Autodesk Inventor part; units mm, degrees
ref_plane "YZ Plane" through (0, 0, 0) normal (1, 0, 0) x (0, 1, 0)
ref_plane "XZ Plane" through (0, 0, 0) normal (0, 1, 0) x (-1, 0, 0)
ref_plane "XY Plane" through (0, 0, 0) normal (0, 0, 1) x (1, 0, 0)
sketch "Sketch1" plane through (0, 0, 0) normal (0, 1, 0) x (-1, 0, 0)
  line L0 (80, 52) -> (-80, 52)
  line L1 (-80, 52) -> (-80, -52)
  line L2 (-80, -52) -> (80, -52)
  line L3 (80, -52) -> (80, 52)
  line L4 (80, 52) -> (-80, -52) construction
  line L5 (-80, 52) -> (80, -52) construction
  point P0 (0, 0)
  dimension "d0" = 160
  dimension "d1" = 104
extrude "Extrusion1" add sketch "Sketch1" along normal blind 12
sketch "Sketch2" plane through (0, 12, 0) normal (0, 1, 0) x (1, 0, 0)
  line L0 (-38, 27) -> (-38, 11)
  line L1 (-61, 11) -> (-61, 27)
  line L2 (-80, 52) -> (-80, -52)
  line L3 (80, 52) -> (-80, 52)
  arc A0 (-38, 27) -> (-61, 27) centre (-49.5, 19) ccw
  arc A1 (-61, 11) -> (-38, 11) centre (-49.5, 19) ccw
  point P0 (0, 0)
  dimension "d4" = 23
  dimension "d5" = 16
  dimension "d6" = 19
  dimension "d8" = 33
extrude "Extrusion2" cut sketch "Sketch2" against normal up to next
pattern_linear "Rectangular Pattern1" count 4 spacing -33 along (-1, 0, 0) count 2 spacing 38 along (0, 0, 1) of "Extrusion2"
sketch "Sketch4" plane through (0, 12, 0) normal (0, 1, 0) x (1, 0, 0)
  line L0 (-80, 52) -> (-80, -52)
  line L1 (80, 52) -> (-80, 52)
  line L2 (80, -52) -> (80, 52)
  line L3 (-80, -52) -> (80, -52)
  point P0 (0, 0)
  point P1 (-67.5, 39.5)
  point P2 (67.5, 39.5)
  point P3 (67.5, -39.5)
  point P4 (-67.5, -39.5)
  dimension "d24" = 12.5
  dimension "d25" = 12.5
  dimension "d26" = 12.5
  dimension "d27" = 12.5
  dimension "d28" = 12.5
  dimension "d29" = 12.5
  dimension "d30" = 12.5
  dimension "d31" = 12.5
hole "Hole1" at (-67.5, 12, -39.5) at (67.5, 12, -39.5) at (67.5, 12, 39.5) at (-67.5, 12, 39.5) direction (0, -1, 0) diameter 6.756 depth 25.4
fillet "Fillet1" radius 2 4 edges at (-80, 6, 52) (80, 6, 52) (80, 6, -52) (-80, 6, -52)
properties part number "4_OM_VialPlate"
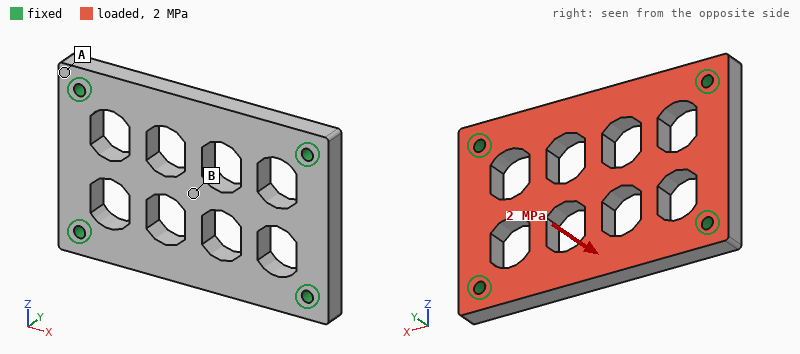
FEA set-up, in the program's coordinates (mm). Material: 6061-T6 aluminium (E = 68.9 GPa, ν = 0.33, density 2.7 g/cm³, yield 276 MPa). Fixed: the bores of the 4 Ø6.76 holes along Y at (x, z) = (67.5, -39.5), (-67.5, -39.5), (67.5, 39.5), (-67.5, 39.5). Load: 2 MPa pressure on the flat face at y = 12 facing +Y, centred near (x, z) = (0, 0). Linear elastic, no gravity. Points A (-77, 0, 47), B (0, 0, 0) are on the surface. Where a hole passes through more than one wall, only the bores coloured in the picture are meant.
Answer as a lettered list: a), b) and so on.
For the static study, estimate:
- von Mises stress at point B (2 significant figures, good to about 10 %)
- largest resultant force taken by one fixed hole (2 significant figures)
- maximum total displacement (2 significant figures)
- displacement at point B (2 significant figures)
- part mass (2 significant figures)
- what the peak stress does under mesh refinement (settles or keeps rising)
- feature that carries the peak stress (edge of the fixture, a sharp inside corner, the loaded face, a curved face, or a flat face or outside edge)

a) 58 MPa
b) 6.0 kN
c) 0.29 mm
d) 0.29 mm
e) 390 g
f) keeps rising
g) edge of the fixture
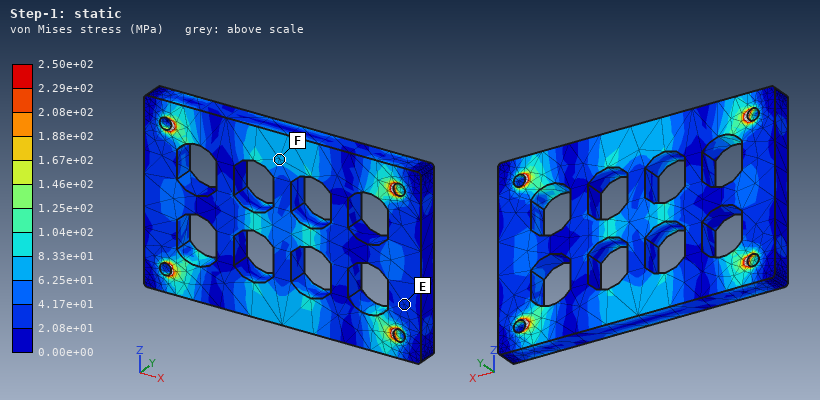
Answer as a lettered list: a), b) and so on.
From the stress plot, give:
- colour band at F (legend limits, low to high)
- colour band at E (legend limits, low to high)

a) 6.25e+01 to 8.33e+01 MPa
b) 2.08e+01 to 4.17e+01 MPa
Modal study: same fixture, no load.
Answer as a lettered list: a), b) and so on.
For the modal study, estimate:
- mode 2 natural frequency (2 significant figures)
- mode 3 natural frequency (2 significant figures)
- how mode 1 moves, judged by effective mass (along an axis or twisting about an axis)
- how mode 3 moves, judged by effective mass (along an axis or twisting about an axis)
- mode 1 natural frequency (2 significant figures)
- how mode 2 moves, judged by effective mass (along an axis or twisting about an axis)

a) 3700 Hz
b) 5800 Hz
c) along Y
d) along Z
e) 2700 Hz
f) twisting about X
